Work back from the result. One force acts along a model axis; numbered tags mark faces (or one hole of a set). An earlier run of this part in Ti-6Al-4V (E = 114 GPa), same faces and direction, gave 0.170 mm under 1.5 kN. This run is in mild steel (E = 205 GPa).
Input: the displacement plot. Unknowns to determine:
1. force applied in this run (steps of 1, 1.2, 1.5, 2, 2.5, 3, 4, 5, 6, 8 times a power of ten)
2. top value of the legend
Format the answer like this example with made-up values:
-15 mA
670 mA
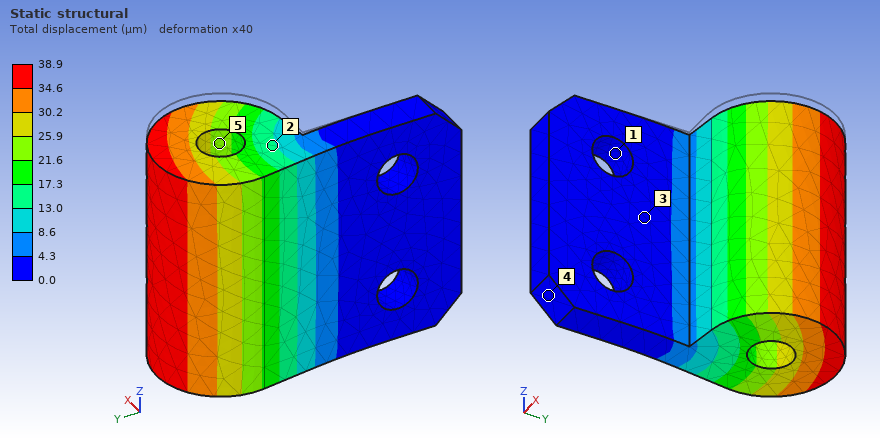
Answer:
600 N
38.9 µm
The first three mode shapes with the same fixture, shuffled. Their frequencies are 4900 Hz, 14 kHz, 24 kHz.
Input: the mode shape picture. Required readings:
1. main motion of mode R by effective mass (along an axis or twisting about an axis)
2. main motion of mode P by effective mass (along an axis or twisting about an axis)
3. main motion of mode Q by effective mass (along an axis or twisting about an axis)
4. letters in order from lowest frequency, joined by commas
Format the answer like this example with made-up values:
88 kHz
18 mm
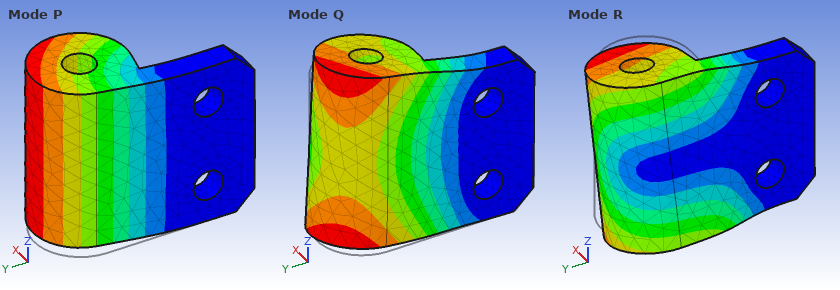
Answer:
along Z
along X
along Z
P, R, Q
